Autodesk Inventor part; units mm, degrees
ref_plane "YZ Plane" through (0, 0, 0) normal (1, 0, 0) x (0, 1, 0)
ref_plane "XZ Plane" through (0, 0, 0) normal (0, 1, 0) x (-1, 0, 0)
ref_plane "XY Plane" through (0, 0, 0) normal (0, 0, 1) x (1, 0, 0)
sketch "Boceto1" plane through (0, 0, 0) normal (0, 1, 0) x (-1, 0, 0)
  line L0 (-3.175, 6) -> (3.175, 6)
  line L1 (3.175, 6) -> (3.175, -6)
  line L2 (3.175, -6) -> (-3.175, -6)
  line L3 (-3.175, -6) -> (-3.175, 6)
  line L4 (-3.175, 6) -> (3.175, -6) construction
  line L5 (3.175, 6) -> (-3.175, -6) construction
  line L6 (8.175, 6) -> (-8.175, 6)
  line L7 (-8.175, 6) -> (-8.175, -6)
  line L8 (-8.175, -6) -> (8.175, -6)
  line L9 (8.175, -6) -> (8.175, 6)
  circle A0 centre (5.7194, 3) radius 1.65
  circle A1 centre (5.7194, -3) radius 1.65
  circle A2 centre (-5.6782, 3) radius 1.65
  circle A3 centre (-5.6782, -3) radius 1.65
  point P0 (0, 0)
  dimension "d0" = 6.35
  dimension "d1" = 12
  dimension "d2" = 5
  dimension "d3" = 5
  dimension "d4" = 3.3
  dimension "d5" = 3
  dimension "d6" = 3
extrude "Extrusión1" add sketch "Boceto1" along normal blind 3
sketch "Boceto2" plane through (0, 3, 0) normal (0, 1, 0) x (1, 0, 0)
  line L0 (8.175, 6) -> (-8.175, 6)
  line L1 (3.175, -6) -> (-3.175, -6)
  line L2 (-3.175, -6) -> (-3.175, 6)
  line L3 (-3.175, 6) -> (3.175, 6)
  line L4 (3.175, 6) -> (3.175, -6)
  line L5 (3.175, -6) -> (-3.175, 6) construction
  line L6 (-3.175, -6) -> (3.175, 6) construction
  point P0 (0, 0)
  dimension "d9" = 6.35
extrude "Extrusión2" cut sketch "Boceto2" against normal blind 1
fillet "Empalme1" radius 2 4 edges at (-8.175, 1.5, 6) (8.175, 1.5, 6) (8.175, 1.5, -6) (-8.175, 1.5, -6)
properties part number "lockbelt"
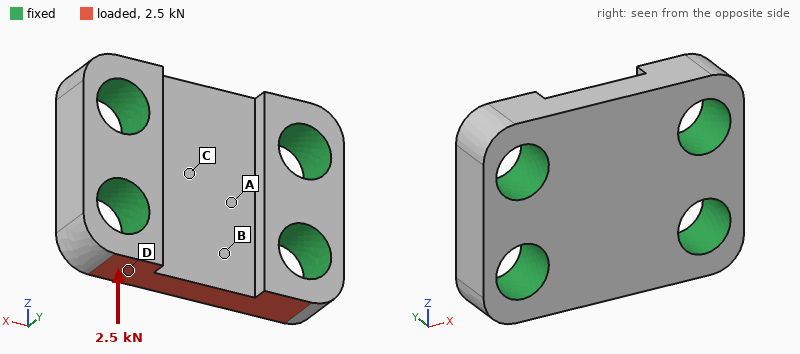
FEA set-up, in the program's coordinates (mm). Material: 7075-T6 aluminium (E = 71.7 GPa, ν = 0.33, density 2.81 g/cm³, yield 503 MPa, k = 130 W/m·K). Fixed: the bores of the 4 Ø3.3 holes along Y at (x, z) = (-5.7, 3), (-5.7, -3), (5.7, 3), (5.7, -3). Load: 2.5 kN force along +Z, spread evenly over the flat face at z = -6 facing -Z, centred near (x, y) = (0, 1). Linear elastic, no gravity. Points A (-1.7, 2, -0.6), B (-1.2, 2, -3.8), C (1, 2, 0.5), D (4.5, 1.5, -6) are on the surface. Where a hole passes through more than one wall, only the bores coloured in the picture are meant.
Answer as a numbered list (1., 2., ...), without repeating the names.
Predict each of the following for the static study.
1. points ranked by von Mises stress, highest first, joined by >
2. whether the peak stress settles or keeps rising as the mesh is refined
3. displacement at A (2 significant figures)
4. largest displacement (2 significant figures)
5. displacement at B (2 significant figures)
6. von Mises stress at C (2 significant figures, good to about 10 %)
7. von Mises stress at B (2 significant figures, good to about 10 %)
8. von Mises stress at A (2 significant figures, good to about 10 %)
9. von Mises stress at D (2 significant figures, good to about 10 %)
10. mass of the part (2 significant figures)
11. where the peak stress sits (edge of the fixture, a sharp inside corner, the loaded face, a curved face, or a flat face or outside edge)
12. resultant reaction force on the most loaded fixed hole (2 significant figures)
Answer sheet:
1. D > B > A > C
2. keeps rising
3. 2.2 µm
4. 7.2 µm
5. 4.5 µm
6. 29 MPa
7. 60 MPa
8. 41 MPa
9. 89 MPa
10. 1.1 g
11. edge of the fixture
12. 1.0 kN
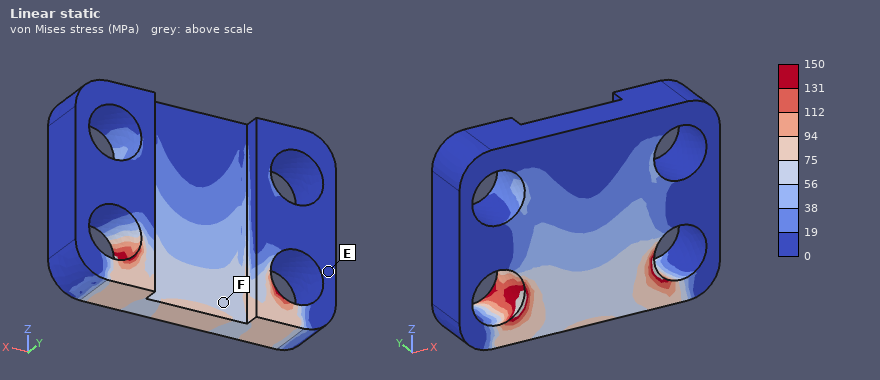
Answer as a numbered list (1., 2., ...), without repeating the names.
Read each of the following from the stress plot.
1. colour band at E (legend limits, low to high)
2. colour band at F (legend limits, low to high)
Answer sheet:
1. 0 to 19 MPa
2. 56 to 75 MPa
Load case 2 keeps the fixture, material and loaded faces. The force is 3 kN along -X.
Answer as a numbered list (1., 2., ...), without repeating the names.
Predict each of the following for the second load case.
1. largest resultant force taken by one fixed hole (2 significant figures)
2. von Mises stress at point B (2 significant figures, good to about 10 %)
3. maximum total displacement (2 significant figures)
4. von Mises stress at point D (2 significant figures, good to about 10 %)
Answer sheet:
1. 1.5 kN
2. 97 MPa
3. 10 µm
4. 190 MPa
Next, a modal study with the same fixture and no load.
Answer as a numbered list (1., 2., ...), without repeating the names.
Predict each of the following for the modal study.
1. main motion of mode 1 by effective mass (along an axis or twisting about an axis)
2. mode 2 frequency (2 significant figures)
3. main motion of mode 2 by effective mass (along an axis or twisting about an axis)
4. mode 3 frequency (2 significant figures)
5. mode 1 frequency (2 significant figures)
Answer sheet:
1. along Y
2. 120 kHz
3. twisting about X
4. 150 kHz
5. 120 kHz
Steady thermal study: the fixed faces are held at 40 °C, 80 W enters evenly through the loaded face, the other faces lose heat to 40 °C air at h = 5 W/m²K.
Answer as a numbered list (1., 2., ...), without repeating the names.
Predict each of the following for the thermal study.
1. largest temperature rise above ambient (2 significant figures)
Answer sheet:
1. 71 K
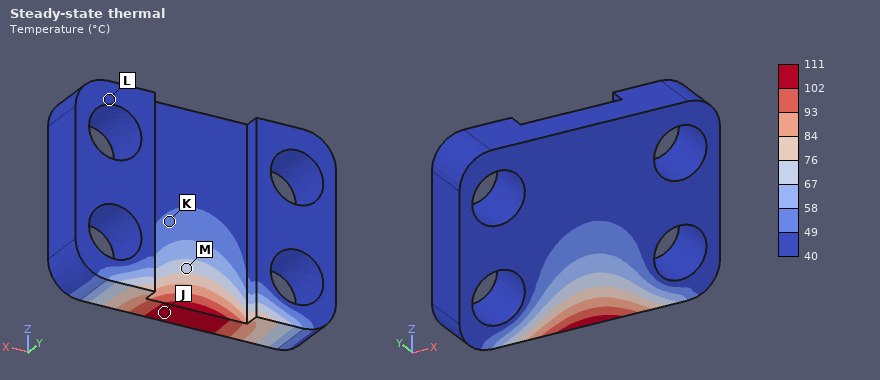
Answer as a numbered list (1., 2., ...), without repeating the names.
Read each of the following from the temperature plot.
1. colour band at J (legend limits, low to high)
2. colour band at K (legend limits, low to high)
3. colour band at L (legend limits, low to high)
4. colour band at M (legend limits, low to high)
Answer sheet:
1. 102 to 111 °C
2. 49 to 58 °C
3. 40 to 49 °C
4. 67 to 76 °C
